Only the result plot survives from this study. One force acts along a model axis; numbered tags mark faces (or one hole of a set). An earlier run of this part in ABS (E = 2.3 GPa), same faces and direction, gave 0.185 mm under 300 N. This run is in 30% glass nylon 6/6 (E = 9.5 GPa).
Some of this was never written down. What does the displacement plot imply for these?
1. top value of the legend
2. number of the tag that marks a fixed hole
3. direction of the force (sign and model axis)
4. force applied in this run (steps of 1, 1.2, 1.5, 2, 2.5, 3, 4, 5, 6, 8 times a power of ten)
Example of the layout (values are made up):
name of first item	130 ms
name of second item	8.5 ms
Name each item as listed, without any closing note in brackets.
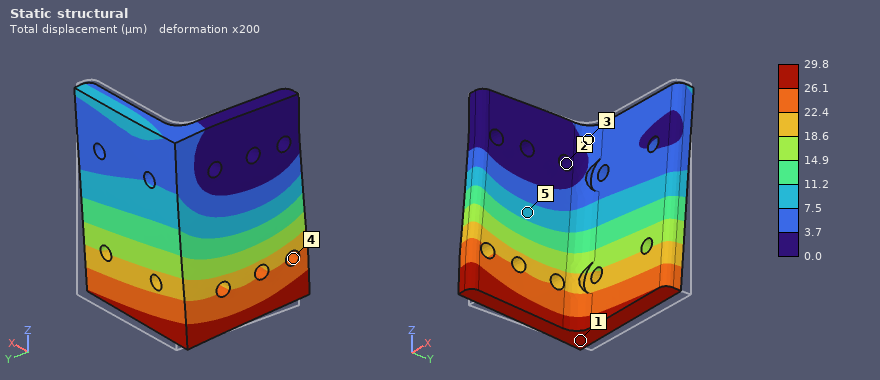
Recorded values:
top value of the legend	29.8 µm
number of the tag that marks a fixed hole	2
direction of the force	-Y
force applied in this run	200 N
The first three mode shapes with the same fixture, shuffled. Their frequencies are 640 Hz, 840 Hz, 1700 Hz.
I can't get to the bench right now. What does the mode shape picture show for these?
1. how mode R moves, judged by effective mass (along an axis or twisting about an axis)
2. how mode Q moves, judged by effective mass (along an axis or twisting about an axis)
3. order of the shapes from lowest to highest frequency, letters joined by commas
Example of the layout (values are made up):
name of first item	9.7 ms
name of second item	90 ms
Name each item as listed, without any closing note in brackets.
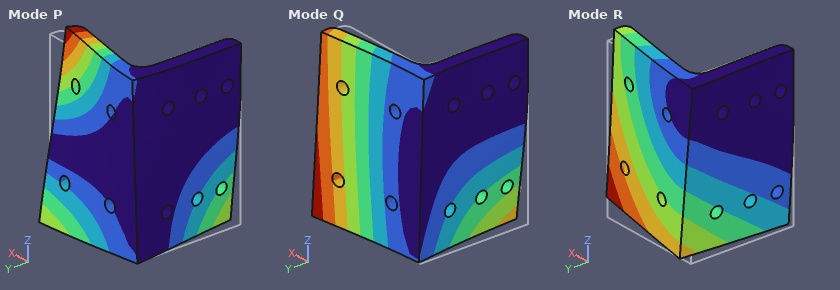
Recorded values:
how mode R moves, judged by effective mass	along X
how mode Q moves, judged by effective mass	along Y
order of the shapes from lowest to highest frequency, letters joined by commas	R, Q, P
